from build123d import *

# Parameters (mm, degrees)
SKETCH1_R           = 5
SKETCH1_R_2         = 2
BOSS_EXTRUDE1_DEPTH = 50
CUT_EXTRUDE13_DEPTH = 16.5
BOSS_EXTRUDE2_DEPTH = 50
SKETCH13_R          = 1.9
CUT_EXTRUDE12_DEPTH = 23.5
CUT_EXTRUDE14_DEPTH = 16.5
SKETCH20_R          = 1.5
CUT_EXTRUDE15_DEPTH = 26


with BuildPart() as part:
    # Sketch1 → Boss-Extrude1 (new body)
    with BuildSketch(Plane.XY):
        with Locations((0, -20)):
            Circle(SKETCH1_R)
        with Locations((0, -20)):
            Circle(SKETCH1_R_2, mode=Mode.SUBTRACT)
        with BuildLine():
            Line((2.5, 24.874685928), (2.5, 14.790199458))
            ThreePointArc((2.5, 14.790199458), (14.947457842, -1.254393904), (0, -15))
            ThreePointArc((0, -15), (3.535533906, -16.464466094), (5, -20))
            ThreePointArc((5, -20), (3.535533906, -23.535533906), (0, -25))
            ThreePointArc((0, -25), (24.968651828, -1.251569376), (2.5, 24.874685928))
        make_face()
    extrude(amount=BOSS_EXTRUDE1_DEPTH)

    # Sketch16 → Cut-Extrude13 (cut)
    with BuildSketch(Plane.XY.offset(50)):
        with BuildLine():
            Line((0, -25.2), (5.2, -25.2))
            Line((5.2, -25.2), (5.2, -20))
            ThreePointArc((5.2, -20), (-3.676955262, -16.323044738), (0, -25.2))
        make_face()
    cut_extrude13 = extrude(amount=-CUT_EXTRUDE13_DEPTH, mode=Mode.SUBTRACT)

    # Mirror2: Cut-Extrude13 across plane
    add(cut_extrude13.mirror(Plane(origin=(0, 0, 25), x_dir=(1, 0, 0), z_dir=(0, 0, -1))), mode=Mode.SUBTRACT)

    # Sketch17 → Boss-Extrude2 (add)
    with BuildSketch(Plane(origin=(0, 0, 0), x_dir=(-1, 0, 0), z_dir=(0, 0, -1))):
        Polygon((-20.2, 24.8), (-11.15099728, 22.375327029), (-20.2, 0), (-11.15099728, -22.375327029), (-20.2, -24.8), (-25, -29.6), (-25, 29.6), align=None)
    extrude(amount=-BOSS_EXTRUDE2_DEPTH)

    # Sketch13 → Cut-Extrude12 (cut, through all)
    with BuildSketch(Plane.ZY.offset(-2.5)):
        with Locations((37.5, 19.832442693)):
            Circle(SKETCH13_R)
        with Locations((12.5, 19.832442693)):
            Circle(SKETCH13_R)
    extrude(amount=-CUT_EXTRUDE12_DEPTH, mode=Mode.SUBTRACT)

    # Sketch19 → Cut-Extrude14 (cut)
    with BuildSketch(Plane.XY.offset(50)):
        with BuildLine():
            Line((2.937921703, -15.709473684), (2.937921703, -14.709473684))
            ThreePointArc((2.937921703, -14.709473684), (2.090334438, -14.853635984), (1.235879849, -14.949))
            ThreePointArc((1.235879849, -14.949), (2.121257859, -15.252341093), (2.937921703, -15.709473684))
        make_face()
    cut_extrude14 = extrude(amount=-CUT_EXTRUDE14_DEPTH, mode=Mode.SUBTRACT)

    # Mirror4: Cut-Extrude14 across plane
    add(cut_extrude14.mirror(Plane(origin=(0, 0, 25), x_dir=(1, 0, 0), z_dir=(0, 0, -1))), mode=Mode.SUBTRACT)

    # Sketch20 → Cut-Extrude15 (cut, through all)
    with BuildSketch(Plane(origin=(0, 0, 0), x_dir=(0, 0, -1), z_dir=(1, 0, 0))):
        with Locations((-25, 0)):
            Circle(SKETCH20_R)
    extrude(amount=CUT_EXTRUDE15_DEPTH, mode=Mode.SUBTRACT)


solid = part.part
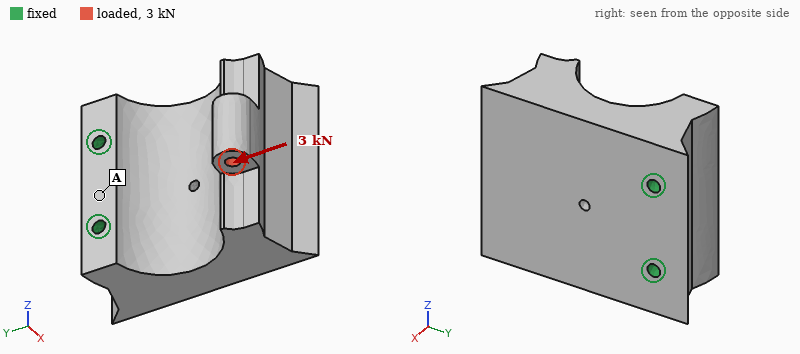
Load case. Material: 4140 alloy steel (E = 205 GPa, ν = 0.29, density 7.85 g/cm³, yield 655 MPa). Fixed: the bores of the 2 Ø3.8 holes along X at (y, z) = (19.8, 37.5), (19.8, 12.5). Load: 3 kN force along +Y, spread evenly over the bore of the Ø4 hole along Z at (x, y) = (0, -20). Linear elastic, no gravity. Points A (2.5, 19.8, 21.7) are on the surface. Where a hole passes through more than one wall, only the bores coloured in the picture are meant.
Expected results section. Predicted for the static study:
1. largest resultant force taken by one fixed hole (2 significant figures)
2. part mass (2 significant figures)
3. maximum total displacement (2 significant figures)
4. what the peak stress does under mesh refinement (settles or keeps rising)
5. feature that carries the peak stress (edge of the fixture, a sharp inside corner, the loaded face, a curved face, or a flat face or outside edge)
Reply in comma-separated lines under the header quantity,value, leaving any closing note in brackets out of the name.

quantity,value
largest resultant force taken by one fixed hole,1.5 kN
part mass,320 g
maximum total displacement,61 µm
what the peak stress does under mesh refinement,keeps rising
feature that carries the peak stress,a sharp inside corner
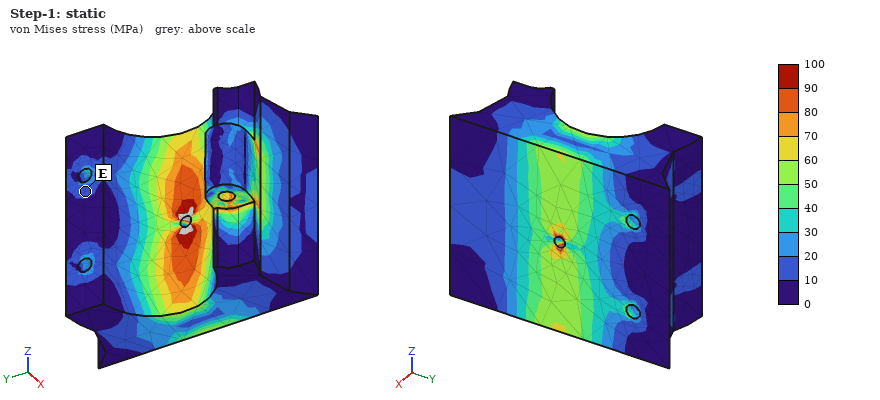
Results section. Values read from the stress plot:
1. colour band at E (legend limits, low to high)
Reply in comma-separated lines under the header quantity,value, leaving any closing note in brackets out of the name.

quantity,value
colour band at E,10 to 20 MPa
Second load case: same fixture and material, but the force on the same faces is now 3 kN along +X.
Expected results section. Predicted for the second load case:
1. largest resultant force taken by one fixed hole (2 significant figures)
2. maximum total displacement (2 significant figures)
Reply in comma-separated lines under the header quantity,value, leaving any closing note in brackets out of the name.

quantity,value
largest resultant force taken by one fixed hole,1.5 kN
maximum total displacement,62 µm
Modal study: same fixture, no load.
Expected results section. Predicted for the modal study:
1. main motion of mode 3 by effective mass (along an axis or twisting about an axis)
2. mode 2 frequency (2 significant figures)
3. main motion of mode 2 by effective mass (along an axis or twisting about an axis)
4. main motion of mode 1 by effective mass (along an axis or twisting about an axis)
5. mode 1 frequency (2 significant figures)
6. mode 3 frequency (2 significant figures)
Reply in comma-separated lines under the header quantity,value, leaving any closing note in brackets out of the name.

quantity,value
main motion of mode 3 by effective mass,along Z
mode 2 frequency,7200 Hz
main motion of mode 2 by effective mass,along Z
main motion of mode 1 by effective mass,along X
mode 1 frequency,3900 Hz
mode 3 frequency,9400 Hz
